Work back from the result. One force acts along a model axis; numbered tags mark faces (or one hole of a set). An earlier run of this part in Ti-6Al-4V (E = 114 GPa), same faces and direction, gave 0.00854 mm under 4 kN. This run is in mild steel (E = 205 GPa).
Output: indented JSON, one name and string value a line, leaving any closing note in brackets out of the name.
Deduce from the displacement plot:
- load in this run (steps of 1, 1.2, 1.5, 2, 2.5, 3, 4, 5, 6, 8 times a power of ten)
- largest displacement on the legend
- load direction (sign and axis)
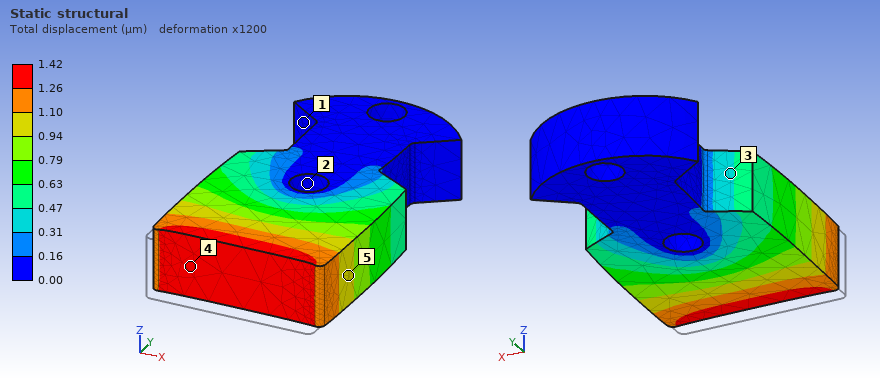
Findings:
{
  "load in this run": "1.2 kN",
  "largest displacement on the legend": "1.42 µm",
  "load direction": "+Y"
}
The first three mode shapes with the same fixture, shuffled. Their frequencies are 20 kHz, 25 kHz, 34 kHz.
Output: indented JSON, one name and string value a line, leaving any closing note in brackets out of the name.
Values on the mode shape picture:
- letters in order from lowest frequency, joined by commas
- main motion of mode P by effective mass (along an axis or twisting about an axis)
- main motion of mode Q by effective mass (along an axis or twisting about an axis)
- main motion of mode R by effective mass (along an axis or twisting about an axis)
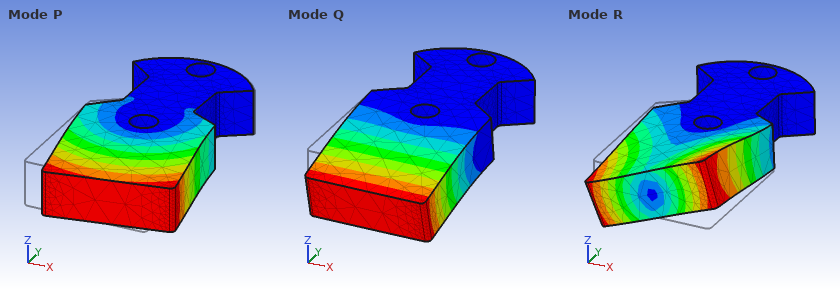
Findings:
{
  "letters in order from lowest frequency, joined by commas": "Q, P, R",
  "main motion of mode P by effective mass": "along X",
  "main motion of mode Q by effective mass": "along Z",
  "main motion of mode R by effective mass": "twisting about Y"
}
